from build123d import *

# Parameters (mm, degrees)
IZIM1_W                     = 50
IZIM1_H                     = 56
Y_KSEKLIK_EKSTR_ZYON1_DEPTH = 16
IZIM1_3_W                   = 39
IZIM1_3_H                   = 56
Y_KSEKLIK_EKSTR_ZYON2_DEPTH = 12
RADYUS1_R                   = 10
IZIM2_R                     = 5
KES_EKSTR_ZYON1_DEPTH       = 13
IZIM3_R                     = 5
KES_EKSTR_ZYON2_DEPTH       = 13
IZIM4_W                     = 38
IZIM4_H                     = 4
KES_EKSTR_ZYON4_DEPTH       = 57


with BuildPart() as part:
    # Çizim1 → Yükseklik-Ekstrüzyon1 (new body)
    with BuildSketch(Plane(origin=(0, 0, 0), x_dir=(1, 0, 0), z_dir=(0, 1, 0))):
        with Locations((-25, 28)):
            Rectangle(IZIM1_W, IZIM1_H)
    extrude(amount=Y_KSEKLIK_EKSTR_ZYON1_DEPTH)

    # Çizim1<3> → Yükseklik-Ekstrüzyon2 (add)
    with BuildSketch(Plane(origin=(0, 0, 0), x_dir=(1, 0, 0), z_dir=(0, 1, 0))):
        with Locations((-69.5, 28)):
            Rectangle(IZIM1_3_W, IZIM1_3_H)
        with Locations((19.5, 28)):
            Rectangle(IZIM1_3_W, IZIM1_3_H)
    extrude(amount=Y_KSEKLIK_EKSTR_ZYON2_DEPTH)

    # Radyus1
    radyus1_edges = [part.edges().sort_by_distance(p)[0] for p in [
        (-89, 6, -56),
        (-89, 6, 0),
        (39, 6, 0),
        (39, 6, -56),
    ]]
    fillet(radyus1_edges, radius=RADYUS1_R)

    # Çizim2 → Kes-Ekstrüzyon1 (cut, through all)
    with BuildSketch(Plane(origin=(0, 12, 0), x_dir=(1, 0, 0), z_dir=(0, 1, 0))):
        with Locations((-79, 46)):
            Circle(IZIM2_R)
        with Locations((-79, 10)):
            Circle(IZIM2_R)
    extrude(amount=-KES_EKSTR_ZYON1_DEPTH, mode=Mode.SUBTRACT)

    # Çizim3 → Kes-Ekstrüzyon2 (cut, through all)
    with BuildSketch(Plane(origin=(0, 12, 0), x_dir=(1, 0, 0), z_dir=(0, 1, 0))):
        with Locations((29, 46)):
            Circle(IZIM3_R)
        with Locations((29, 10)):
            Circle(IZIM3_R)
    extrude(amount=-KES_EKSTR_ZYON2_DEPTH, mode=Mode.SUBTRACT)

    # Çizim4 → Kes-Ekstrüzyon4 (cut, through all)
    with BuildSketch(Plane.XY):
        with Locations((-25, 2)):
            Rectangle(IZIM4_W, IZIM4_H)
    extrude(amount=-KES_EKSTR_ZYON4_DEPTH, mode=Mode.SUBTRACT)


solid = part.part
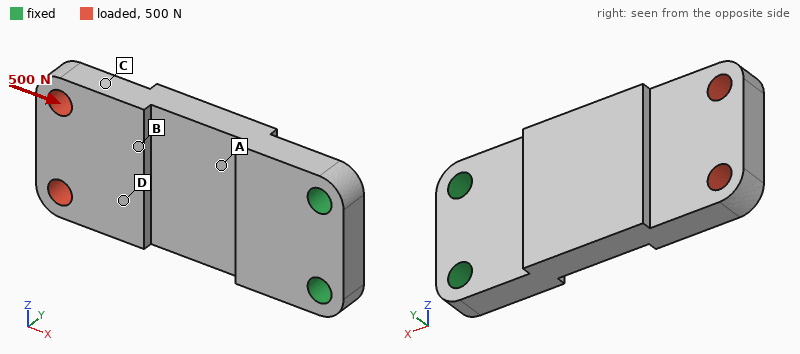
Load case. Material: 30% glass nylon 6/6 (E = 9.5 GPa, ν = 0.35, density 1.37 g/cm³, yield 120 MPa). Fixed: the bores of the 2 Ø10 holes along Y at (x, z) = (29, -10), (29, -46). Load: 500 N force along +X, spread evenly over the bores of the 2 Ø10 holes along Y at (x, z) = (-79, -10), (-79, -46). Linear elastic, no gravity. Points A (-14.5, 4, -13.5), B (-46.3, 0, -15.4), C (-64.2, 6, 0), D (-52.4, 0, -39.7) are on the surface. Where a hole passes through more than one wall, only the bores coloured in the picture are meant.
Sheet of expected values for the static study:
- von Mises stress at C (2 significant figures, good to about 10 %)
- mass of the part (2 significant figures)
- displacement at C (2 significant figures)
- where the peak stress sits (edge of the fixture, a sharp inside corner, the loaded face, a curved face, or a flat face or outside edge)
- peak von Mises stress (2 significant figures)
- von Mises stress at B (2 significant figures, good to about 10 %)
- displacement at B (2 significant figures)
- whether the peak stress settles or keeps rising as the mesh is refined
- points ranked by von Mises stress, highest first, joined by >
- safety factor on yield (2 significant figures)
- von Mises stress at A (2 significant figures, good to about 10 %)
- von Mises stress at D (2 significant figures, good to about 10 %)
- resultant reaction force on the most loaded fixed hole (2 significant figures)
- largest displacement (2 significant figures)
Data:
1.1 MPa
110 g
48 µm
the loaded face
2.7 MPa
0.45 MPa
31 µm
settles
A > C > D > B
44
2.1 MPa
0.72 MPa
250 N
79 µm
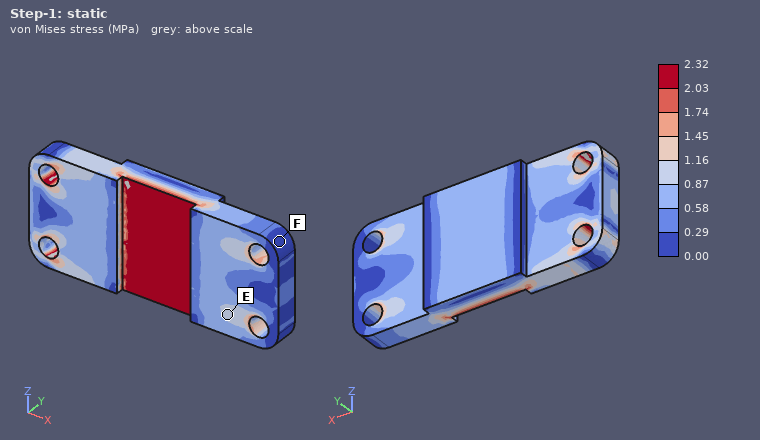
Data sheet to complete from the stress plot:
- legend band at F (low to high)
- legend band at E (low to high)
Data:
0.00 to 0.29 MPa
0.87 to 1.16 MPa
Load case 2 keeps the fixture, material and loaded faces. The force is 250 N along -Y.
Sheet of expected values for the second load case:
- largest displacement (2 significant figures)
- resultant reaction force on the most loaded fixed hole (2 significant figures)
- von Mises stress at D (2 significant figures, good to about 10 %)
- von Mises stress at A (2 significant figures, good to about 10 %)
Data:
1.5 mm
130 N
4.3 MPa
12 MPa
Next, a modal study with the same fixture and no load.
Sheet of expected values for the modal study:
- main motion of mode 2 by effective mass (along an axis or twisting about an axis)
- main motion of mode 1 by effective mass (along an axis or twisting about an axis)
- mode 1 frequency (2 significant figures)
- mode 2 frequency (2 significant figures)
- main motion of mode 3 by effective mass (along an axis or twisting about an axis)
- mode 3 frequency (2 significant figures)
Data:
along Z
along Y
390 Hz
1400 Hz
along Z
1700 Hz
